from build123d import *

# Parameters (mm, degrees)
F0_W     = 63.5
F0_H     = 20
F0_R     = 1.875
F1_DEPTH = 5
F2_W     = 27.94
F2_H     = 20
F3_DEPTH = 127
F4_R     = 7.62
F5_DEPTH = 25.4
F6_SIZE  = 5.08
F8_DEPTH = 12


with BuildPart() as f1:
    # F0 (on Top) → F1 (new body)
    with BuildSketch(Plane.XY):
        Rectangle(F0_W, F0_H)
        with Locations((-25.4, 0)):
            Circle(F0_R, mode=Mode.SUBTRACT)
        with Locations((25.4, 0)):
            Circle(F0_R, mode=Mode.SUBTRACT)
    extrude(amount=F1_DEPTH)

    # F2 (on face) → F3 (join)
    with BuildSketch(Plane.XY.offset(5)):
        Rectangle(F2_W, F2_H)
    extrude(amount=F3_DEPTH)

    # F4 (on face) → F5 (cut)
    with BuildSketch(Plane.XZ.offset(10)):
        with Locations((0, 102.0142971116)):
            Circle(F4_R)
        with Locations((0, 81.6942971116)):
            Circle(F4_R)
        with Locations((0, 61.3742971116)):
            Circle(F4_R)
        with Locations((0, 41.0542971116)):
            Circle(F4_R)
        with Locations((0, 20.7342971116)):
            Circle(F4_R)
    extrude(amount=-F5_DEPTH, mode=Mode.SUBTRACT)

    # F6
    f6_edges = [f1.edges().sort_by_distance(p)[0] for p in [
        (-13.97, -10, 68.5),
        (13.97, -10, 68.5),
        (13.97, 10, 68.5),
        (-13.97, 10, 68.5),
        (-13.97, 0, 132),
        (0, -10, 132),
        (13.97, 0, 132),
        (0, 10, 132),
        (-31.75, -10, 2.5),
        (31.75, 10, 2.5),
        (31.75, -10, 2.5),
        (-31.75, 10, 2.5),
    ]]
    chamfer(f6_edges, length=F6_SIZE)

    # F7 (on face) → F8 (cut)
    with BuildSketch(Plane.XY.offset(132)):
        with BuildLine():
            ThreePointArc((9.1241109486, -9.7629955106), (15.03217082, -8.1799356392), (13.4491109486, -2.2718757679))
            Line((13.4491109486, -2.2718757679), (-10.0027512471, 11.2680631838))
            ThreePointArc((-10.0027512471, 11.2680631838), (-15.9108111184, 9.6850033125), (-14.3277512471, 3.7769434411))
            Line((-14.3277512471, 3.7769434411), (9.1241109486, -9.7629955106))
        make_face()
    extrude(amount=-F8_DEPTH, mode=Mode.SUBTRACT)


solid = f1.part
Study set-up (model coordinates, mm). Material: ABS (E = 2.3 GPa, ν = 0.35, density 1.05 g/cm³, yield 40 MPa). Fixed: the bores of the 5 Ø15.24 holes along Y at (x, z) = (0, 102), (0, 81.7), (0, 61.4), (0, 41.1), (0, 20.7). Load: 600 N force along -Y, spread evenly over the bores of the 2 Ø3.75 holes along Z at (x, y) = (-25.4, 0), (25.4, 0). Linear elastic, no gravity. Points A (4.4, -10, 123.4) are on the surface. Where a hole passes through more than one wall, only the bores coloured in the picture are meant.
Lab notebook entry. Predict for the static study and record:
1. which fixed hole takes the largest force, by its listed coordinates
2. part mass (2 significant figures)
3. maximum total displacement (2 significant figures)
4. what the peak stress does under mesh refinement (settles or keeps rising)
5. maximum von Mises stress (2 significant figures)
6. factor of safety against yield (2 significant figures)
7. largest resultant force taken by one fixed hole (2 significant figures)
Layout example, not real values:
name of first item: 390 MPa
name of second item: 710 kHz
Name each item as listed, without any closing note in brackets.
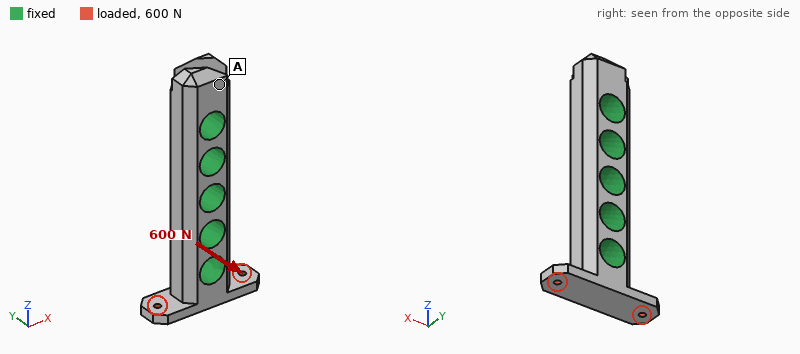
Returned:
which fixed hole takes the largest force, by its listed coordinates: (0, 20.7)
part mass: 51 g
maximum total displacement: 0.25 mm
what the peak stress does under mesh refinement: settles
maximum von Mises stress: 15 MPa
factor of safety against yield: 2.7
largest resultant force taken by one fixed hole: 600 N
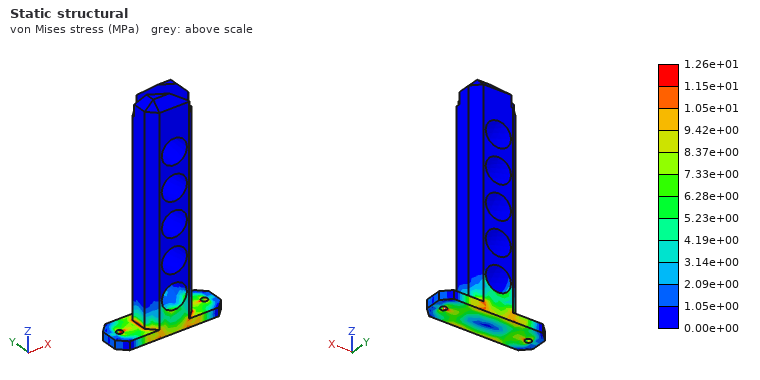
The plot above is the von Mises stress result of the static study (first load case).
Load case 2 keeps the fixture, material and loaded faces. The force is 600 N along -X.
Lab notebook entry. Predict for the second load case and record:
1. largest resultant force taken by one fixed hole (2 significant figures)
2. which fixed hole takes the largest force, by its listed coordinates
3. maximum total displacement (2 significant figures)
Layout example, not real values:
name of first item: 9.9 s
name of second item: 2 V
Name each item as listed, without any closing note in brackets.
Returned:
largest resultant force taken by one fixed hole: 650 N
which fixed hole takes the largest force, by its listed coordinates: (0, 20.7)
maximum total displacement: 0.11 mm
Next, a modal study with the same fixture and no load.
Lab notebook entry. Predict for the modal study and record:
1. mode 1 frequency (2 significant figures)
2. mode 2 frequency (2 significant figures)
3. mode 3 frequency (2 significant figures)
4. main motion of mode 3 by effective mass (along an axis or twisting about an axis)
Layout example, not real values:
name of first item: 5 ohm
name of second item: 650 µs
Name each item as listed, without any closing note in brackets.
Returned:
mode 1 frequency: 2900 Hz
mode 2 frequency: 3000 Hz
mode 3 frequency: 4500 Hz
main motion of mode 3 by effective mass: twisting about Z
